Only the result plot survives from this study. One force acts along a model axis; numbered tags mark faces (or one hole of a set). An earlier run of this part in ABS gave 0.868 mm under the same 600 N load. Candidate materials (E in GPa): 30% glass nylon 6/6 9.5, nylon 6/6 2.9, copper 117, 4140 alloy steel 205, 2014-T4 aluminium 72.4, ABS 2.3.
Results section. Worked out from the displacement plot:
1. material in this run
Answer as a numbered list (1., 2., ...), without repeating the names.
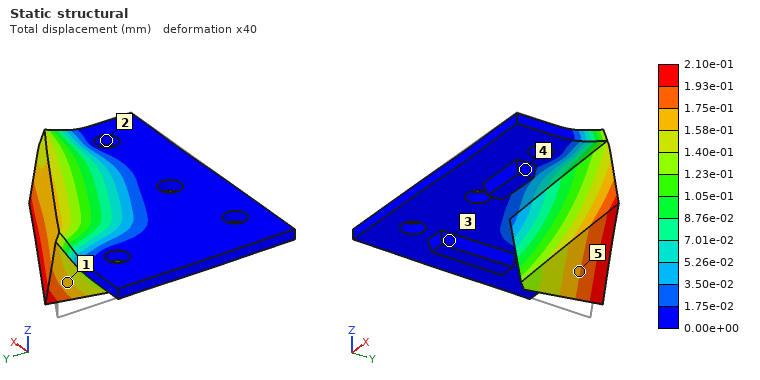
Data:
1. 30% glass nylon 6/6
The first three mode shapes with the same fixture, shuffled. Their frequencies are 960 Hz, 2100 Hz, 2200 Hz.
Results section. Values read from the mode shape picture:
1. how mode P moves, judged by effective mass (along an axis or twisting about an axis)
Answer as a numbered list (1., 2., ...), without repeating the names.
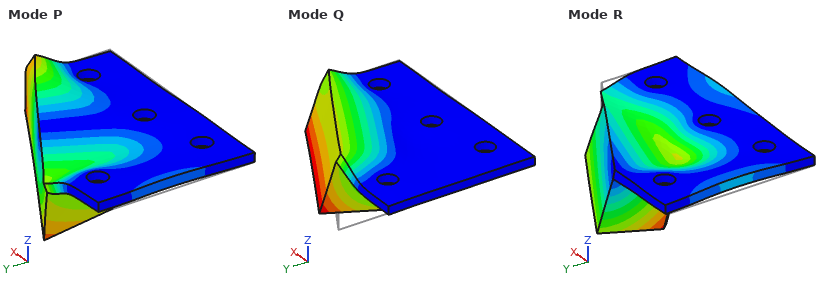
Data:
1. along X
